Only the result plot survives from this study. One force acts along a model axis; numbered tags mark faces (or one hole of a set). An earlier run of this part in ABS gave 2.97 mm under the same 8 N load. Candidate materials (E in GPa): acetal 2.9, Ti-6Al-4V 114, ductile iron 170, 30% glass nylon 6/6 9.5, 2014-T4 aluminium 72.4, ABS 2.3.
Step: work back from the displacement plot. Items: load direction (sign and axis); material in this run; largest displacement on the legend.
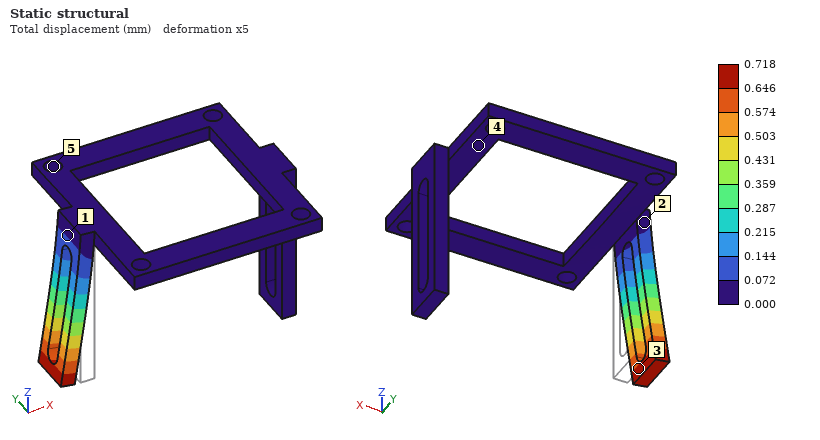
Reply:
-X
30% glass nylon 6/6
0.718 mm
